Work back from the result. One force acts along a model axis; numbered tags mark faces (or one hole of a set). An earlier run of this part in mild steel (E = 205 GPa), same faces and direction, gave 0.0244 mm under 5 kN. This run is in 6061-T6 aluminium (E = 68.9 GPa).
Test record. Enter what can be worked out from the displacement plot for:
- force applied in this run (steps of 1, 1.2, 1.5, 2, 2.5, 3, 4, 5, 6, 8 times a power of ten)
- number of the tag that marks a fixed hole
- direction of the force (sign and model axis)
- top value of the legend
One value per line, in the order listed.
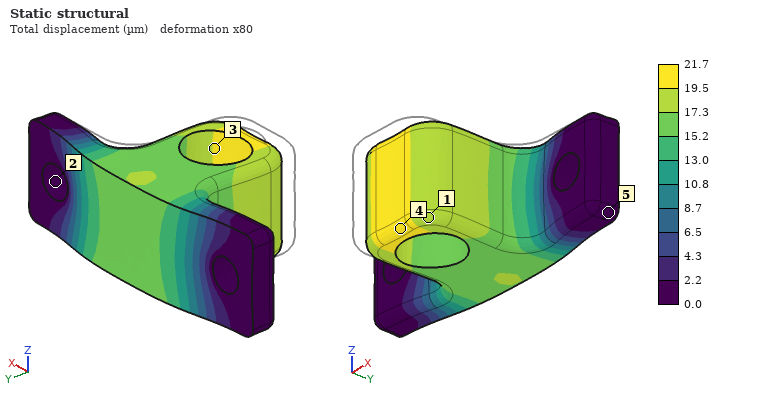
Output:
1.5 kN
2
+Y
21.7 µm
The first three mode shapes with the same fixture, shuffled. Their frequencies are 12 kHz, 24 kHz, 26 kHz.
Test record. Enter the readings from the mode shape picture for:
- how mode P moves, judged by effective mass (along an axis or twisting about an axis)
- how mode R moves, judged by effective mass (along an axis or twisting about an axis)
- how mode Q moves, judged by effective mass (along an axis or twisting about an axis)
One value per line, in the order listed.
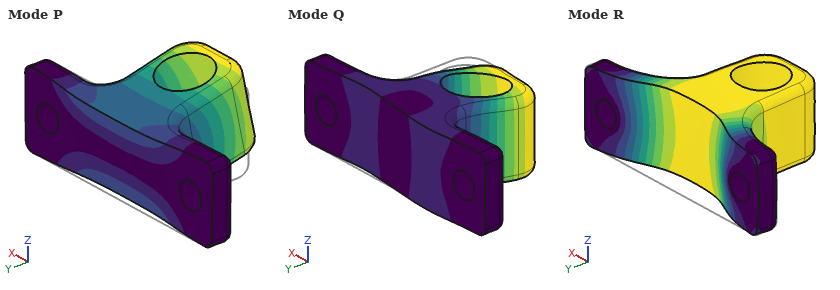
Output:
along Z
along Y
along X
